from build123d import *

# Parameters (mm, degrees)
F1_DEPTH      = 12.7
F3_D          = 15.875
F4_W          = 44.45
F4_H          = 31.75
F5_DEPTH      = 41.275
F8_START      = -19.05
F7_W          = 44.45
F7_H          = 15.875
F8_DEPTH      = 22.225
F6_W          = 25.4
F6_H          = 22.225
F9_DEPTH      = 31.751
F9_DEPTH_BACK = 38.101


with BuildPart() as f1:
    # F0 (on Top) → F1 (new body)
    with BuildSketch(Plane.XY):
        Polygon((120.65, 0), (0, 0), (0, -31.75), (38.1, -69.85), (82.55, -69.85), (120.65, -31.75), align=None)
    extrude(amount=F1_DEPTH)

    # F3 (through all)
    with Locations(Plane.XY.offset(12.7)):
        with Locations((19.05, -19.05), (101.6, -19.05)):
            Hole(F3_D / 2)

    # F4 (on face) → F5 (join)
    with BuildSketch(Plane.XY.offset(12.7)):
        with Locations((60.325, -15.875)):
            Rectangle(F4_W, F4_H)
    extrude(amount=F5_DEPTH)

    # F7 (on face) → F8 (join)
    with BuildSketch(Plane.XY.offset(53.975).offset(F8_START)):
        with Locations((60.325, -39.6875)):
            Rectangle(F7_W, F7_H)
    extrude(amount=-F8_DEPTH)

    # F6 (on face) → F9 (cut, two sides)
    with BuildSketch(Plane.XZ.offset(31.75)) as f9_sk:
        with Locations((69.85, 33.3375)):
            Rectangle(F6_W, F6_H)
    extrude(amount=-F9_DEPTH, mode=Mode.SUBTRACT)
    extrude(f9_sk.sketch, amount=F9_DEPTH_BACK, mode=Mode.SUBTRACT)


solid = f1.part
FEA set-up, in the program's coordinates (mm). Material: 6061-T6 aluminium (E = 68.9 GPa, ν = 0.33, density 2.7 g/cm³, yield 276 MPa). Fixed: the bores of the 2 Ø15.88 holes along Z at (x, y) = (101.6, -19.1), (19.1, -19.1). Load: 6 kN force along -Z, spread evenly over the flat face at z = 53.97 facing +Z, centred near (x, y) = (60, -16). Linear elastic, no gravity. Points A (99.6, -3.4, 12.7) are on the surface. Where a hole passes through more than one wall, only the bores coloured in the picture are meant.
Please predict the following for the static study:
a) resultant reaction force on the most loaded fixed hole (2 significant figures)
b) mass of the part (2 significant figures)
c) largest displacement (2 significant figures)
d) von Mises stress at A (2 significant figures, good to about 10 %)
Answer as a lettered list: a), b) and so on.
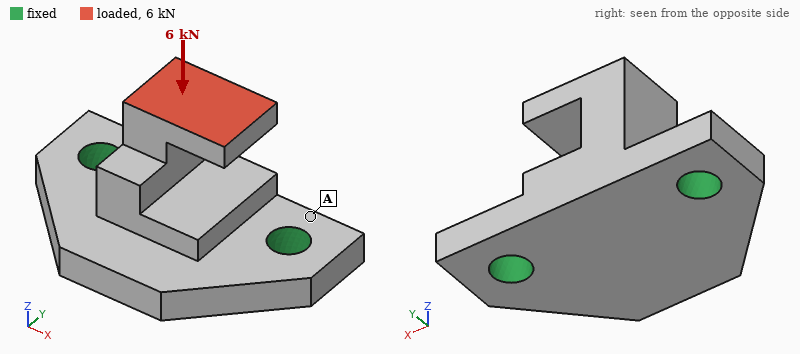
a) 3.5 kN
b) 360 g
c) 0.19 mm
d) 10 MPa
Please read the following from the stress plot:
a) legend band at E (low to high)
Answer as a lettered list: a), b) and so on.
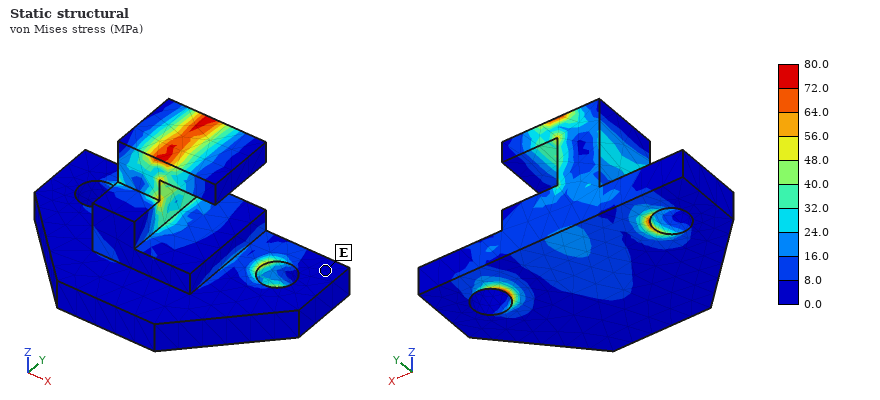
a) 0.0 to 8.0 MPa
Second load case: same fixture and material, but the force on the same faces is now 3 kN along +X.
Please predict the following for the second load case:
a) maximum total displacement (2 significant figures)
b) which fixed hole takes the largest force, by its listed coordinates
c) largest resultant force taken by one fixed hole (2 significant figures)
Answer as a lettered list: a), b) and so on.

a) 0.11 mm
b) (101.6, -19.1)
c) 3.2 kN
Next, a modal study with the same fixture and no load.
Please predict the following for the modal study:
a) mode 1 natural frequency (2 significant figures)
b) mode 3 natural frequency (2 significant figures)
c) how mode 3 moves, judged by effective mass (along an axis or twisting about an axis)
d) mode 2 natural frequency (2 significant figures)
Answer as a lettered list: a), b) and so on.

a) 3400 Hz
b) 6800 Hz
c) along Z
d) 4800 Hz
